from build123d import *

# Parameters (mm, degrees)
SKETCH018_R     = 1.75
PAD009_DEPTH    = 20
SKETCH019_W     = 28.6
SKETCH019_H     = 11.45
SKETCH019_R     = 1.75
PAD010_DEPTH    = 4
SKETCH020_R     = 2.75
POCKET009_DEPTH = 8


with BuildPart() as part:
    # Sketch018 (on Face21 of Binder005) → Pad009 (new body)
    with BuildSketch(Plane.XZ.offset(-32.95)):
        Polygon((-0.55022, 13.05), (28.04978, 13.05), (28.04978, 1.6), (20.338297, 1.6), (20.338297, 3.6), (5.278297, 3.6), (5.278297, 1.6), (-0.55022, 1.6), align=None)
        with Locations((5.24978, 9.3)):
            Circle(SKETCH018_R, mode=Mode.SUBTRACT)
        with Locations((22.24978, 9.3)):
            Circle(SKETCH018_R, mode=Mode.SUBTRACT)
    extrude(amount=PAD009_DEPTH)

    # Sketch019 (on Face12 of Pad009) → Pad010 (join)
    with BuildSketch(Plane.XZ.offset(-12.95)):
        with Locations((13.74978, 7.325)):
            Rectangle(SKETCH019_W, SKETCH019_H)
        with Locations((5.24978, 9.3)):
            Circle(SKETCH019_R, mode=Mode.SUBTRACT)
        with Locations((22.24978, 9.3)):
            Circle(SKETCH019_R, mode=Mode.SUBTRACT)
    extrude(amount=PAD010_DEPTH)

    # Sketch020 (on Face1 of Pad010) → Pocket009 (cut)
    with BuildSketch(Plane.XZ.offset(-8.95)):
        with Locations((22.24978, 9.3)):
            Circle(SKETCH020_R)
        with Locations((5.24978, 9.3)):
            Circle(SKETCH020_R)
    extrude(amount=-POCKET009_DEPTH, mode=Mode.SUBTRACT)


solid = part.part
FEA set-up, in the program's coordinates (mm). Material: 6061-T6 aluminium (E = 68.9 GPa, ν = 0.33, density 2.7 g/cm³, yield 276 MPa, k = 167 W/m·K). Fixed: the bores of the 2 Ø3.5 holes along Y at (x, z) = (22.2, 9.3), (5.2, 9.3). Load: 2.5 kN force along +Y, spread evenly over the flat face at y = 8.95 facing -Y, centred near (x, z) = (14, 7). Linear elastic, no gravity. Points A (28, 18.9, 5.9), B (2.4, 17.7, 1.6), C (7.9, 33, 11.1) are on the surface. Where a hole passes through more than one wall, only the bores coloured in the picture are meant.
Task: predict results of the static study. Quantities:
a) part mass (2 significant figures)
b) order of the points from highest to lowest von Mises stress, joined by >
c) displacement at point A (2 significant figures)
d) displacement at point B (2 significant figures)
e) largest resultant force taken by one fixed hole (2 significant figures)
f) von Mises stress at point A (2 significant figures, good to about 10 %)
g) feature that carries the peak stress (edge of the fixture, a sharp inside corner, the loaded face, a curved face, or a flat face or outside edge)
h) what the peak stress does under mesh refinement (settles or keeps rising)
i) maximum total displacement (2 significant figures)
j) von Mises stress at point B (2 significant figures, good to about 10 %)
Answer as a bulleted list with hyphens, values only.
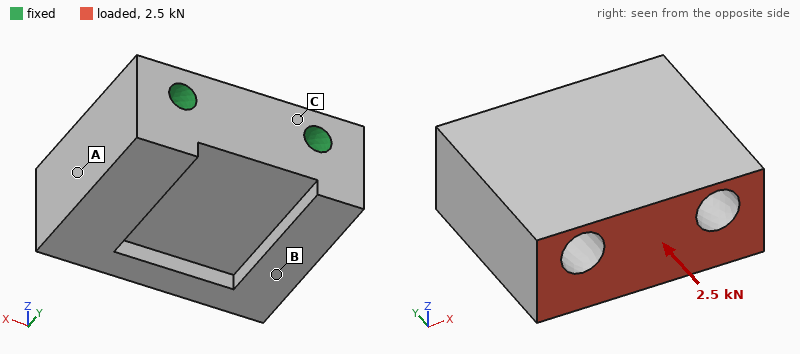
- 18 g
- B > A > C
- 1.2 µm
- 2.1 µm
- 1.3 kN
- 8.0 MPa
- edge of the fixture
- keeps rising
- 5.2 µm
- 12 MPa
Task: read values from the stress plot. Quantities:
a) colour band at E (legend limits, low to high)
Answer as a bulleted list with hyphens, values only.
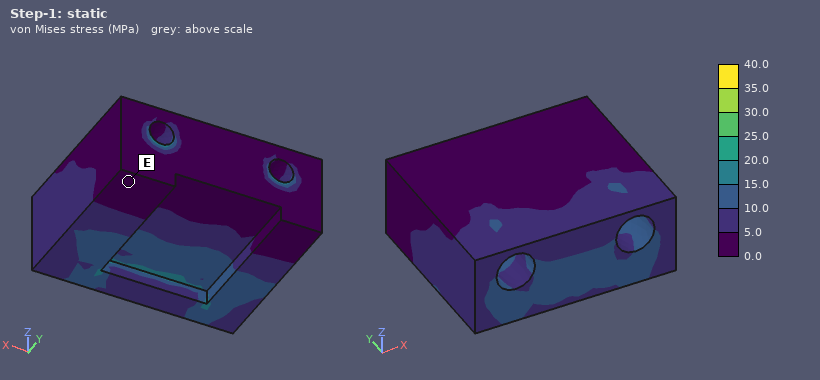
- 0.0 to 5.0 MPa
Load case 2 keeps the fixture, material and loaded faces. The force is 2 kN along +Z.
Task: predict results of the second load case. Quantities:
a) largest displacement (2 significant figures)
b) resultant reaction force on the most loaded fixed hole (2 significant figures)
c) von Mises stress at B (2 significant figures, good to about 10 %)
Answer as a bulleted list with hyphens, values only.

- 21 µm
- 1.0 kN
- 39 MPa
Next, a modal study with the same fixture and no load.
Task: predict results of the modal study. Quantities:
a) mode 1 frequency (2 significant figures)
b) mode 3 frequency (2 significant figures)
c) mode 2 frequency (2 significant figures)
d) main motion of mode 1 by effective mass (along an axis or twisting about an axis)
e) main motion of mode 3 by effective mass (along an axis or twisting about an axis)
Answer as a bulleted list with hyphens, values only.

- 32 kHz
- 49 kHz
- 42 kHz
- along Z
- along X
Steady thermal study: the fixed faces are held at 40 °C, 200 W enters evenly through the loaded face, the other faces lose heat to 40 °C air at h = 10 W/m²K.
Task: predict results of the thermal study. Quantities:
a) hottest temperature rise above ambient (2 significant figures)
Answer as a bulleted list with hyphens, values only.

- 63 K
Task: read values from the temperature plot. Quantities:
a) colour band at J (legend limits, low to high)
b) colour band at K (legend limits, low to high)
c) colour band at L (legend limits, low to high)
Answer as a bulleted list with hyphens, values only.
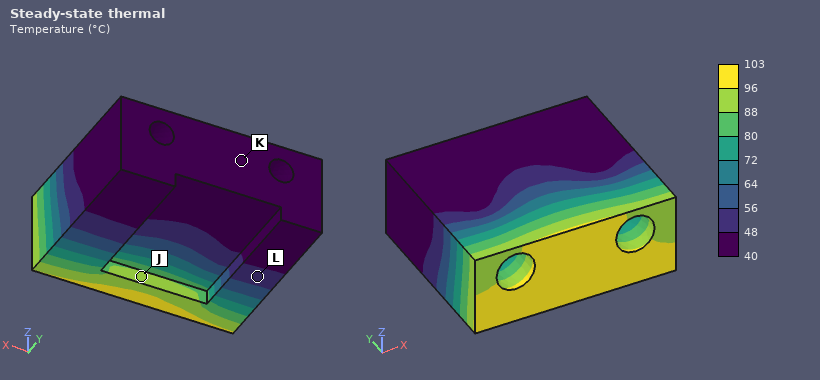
- 88 to 96 °C
- 40 to 48 °C
- 48 to 56 °C
